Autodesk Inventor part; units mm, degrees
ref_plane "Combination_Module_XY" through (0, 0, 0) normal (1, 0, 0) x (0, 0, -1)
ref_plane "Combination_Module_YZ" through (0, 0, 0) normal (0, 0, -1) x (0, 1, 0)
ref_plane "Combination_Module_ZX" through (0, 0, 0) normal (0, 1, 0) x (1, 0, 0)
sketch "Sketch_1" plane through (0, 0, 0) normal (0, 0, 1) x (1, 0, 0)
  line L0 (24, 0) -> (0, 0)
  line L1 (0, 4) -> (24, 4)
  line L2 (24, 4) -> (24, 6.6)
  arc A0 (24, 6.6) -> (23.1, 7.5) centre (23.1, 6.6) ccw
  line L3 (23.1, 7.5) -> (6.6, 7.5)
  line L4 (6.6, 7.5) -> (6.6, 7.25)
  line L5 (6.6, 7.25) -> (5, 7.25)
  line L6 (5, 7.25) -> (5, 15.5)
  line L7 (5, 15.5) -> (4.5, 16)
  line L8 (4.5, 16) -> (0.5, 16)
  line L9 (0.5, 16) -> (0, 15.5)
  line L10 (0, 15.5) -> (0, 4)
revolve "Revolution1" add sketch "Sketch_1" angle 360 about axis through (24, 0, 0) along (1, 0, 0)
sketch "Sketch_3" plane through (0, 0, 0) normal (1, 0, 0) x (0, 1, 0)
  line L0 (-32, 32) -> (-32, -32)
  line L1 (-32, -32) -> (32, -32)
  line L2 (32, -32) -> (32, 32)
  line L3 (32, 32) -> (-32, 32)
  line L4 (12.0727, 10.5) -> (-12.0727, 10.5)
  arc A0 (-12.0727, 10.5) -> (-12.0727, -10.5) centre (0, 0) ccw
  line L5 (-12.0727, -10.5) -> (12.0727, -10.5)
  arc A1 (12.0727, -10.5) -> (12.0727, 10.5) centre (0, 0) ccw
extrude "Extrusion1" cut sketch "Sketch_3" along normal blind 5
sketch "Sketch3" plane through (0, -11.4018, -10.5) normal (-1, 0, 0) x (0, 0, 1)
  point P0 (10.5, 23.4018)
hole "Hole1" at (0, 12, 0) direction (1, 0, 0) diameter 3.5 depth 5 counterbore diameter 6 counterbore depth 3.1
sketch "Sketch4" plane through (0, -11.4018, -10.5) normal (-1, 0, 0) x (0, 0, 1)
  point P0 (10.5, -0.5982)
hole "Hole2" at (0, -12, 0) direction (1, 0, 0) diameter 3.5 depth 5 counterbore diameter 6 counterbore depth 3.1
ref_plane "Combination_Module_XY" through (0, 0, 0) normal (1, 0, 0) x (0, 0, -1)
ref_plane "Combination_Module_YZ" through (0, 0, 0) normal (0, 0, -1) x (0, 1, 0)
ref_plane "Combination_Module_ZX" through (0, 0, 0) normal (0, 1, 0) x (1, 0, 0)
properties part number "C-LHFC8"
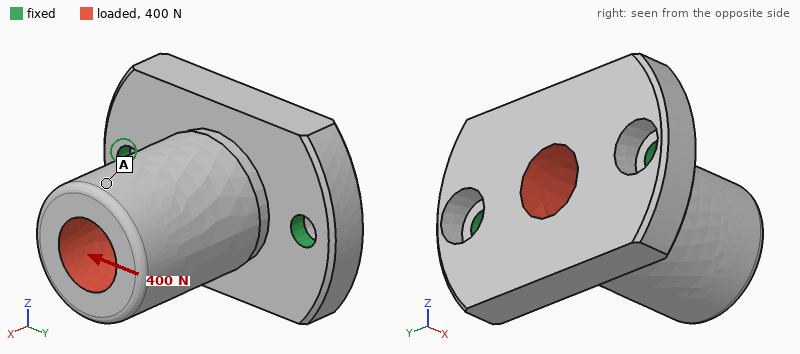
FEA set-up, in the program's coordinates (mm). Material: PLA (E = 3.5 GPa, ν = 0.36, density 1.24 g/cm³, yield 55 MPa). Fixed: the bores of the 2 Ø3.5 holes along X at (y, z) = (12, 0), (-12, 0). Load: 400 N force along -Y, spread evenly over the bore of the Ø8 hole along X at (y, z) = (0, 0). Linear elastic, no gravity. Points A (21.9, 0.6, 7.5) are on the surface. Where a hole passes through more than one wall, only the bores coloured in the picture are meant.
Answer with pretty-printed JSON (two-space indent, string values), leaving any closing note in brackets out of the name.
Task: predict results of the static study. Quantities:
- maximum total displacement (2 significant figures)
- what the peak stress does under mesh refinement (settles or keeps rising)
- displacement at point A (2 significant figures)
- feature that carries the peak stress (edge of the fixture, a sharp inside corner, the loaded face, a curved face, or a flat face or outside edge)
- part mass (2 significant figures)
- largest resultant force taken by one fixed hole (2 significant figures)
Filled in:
{
  "maximum total displacement": "0.19 mm",
  "what the peak stress does under mesh refinement": "keeps rising",
  "displacement at point A": "0.16 mm",
  "feature that carries the peak stress": "edge of the fixture",
  "part mass": "6.2 g",
  "largest resultant force taken by one fixed hole": "250 N"
}
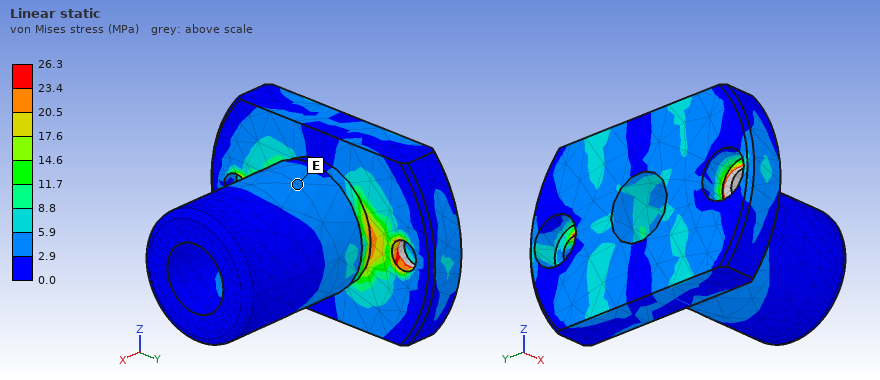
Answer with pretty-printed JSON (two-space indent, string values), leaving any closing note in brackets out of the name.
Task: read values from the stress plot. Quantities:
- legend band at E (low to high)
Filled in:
{
  "legend band at E": "2.9 to 5.9 MPa"
}
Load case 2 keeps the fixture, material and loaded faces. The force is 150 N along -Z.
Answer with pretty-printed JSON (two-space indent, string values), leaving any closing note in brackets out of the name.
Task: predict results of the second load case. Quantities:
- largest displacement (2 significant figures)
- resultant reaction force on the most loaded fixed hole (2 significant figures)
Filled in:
{
  "largest displacement": "0.39 mm",
  "resultant reaction force on the most loaded fixed hole": "75 N"
}
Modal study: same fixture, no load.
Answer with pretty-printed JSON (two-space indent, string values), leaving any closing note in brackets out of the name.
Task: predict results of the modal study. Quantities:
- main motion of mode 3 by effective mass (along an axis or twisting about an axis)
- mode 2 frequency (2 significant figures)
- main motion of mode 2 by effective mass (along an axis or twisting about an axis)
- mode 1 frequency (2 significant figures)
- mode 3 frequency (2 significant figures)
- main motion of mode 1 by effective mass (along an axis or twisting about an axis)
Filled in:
{
  "main motion of mode 3 by effective mass": "along X",
  "mode 2 frequency": "4400 Hz",
  "main motion of mode 2 by effective mass": "along Y",
  "mode 1 frequency": "1700 Hz",
  "mode 3 frequency": "5400 Hz",
  "main motion of mode 1 by effective mass": "along Z"
}
